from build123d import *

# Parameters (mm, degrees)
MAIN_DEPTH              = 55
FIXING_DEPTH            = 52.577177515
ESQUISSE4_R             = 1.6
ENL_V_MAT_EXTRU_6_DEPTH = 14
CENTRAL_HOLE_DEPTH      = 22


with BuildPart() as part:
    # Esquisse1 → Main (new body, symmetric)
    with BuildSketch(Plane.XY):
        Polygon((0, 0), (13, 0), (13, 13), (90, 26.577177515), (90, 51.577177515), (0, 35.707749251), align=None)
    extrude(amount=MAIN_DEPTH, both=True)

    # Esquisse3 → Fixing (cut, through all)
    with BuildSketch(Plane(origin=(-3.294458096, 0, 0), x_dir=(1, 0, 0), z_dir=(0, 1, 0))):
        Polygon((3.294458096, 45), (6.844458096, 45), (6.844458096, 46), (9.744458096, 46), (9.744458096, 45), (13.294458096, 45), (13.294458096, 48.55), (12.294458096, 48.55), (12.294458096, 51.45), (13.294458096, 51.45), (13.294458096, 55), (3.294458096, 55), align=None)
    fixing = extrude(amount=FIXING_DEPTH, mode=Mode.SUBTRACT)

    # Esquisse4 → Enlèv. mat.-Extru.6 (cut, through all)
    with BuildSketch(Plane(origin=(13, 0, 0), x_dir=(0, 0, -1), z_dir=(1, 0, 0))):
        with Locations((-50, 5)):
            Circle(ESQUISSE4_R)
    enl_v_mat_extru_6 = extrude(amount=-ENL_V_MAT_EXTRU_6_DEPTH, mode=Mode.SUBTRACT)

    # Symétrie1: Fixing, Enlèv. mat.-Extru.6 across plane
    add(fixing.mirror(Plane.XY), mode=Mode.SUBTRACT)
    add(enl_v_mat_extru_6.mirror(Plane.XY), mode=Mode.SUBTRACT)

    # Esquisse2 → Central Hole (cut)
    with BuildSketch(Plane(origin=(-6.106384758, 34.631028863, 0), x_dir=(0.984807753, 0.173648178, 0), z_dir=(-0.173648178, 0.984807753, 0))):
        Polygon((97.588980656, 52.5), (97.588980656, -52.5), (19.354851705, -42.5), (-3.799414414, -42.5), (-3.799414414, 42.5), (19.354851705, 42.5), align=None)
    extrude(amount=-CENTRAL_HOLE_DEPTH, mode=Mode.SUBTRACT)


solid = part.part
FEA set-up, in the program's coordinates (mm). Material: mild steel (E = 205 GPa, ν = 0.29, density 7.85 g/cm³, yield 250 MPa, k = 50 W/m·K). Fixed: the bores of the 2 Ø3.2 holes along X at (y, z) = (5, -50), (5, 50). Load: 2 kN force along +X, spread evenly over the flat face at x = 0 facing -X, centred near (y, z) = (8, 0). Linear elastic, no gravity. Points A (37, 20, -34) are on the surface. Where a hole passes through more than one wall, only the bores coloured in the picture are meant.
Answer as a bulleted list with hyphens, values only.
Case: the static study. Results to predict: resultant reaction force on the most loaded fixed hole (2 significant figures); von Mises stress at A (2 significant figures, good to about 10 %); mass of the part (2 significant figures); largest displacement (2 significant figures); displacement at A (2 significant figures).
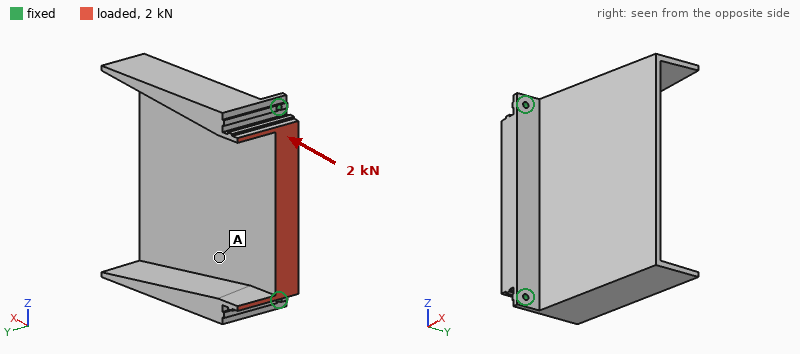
- 1.1 kN
- 6.2 MPa
- 550 g
- 54 µm
- 21 µm
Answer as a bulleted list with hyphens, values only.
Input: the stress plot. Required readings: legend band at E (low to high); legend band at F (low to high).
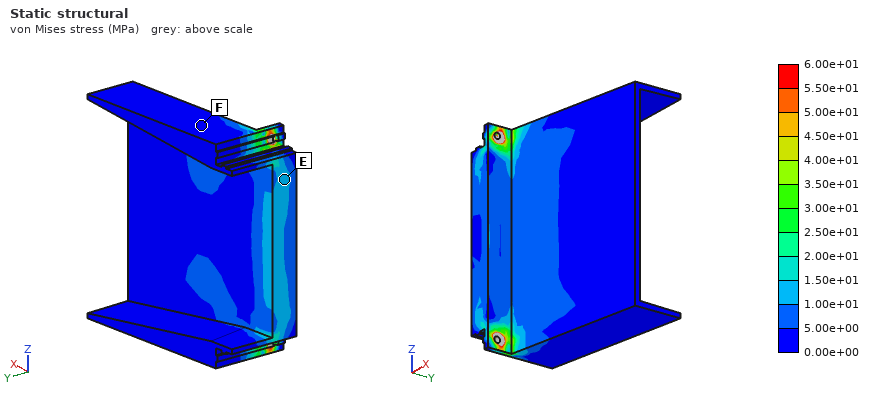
- 1.00e+01 to 1.50e+01 MPa
- 0.00e+00 to 5.00e+00 MPa
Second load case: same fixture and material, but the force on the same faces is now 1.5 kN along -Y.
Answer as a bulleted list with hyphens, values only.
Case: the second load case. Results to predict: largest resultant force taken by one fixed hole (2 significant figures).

- 1.2 kN
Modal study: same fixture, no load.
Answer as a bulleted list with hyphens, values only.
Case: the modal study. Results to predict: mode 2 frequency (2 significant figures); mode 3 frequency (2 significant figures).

- 840 Hz
- 1600 Hz
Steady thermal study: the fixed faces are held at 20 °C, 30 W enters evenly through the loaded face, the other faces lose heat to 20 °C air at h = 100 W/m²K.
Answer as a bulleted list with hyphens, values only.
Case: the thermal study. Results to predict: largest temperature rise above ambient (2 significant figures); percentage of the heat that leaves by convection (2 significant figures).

- 28 K
- 73 %
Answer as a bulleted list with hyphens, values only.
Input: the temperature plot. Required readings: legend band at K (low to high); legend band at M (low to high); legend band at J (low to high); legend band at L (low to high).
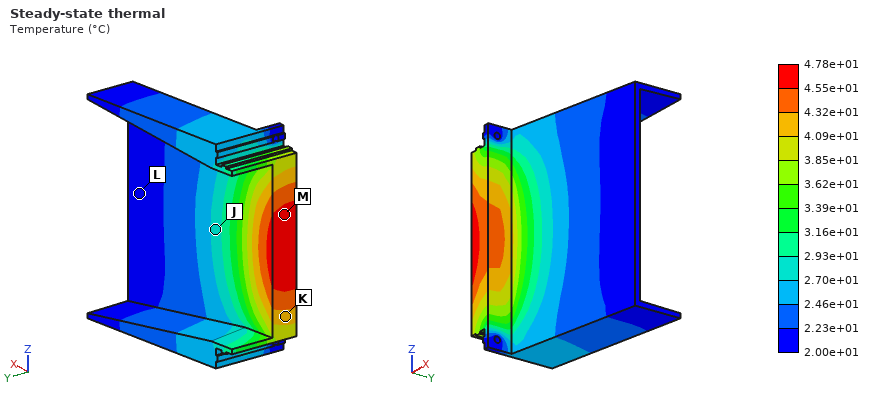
- 4.09e+01 to 4.32e+01 °C
- 4.55e+01 to 4.78e+01 °C
- 2.70e+01 to 2.93e+01 °C
- 2.00e+01 to 2.23e+01 °C
